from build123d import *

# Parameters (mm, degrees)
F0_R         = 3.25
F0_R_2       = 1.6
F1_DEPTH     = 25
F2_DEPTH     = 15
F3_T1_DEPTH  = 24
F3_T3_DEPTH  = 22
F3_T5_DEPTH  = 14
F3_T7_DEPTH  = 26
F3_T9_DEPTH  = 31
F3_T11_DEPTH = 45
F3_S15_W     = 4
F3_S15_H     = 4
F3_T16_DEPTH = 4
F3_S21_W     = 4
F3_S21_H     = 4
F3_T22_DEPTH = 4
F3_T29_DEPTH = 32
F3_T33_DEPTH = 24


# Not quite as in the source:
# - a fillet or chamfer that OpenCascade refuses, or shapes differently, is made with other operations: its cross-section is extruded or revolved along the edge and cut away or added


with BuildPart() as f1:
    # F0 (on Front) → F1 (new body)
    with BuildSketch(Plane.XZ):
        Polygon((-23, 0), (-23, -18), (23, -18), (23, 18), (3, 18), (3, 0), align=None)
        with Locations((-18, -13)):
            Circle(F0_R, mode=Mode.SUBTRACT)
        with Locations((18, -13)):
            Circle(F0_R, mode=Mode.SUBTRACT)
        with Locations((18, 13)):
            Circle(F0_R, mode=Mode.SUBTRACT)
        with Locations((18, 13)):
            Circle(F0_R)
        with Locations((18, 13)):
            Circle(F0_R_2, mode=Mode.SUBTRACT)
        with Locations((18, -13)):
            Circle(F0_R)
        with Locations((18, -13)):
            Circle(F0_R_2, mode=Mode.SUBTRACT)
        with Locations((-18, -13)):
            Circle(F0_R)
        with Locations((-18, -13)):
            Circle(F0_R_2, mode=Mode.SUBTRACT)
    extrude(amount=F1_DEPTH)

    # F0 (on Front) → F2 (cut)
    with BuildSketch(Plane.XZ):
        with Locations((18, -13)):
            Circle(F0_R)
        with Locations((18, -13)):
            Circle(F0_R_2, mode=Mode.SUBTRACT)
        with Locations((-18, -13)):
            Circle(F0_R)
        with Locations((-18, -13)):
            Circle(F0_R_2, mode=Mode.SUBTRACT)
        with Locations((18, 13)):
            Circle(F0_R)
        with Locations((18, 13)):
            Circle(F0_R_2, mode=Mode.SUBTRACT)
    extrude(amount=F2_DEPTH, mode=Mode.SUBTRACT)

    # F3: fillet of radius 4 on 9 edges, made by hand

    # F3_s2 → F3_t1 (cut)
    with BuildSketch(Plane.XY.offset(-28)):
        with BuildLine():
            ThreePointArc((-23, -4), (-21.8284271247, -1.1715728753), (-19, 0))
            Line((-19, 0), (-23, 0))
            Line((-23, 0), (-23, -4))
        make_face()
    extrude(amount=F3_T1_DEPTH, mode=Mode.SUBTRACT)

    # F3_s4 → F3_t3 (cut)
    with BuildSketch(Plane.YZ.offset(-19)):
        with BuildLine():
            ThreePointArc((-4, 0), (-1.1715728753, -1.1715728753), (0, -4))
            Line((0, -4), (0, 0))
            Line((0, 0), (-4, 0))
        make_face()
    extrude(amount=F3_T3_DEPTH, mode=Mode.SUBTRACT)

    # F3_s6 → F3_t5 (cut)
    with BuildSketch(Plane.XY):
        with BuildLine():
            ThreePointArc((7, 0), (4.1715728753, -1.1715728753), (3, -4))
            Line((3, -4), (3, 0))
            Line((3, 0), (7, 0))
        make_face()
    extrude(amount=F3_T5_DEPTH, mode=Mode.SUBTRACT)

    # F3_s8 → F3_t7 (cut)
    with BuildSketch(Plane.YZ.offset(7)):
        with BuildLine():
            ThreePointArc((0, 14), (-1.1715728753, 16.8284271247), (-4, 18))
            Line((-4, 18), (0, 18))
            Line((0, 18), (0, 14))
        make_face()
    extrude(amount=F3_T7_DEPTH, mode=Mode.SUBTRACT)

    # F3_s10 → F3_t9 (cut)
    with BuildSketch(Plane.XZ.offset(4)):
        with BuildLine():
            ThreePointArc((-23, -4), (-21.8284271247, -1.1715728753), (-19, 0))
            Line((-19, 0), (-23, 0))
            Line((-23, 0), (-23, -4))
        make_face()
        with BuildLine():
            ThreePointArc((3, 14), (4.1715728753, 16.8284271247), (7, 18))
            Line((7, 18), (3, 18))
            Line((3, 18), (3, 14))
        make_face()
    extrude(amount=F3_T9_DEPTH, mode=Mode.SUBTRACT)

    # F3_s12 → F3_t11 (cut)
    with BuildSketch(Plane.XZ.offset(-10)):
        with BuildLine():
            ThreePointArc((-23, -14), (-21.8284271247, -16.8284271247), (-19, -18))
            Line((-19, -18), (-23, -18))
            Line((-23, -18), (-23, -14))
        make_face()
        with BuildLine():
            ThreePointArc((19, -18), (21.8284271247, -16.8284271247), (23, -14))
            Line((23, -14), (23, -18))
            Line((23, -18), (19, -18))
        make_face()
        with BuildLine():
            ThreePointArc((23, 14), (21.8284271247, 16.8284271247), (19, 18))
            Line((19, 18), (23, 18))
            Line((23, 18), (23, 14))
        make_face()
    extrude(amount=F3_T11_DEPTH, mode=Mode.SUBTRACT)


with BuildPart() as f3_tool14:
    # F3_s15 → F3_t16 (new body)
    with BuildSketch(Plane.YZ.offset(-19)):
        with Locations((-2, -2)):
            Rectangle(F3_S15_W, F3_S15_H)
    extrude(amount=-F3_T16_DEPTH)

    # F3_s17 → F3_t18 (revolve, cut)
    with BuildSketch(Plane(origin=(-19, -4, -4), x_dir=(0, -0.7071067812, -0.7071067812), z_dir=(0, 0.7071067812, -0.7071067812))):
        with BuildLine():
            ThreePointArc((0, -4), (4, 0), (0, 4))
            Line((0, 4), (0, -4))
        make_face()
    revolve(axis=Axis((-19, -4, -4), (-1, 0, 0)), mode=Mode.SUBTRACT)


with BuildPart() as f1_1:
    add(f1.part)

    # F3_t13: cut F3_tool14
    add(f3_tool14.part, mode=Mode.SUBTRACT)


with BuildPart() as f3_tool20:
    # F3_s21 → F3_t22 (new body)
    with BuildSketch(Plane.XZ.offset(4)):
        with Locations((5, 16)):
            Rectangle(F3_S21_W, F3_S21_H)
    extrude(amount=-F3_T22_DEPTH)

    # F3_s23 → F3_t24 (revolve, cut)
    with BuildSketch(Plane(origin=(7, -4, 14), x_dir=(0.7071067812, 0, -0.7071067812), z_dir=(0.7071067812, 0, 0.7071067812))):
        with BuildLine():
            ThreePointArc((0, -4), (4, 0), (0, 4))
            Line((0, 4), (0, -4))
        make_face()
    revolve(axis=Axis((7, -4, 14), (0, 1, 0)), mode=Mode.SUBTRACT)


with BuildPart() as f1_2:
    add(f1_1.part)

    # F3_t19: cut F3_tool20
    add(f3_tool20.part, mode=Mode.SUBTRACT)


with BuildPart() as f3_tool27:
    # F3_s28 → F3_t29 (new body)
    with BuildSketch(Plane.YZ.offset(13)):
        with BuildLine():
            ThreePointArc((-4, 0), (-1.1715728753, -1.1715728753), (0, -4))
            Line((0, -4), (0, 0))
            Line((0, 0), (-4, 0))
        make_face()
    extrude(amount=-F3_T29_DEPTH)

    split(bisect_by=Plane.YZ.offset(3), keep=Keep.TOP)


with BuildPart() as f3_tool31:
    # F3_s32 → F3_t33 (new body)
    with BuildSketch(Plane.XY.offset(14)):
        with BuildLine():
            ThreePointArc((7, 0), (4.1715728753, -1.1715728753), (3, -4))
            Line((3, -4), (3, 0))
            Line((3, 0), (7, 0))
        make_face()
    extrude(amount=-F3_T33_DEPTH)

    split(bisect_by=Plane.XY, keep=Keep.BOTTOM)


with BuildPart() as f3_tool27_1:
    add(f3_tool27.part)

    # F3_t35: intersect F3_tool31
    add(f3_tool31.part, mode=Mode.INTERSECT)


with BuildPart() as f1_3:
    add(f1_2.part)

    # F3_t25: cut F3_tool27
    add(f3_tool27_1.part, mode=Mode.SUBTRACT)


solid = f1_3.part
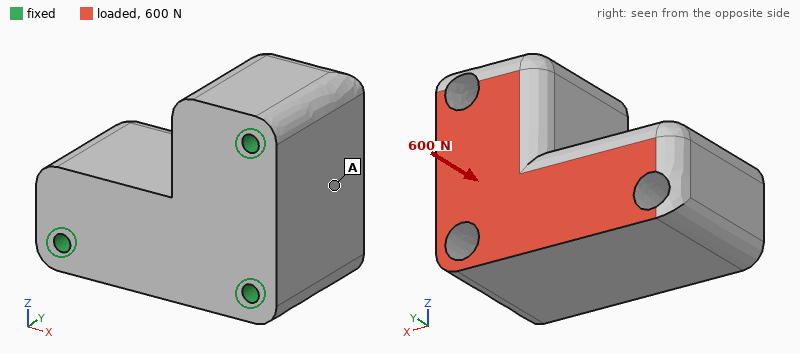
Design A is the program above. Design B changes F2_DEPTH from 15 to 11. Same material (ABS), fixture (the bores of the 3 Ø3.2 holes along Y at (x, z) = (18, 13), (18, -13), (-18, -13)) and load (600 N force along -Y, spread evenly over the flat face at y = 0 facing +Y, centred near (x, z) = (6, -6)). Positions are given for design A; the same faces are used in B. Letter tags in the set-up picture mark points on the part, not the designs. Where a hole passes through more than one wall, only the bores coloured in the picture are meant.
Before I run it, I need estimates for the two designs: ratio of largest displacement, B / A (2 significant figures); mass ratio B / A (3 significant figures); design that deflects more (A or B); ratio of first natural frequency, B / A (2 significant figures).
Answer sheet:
0.82
1.01
A
1.3
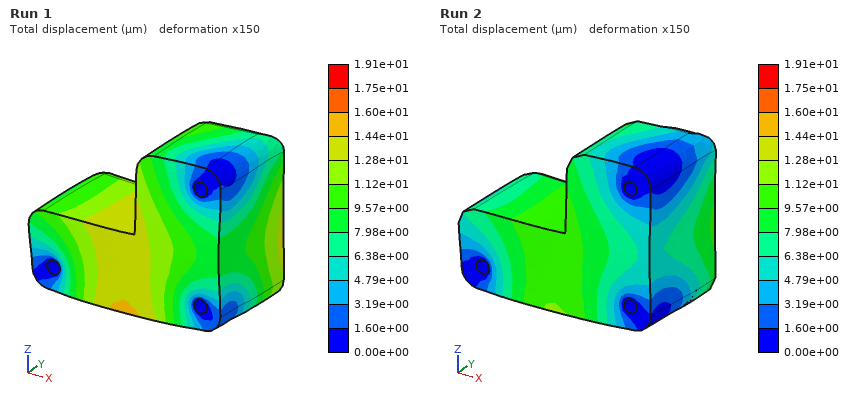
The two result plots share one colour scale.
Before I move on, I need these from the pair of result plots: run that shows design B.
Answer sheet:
Run 2
